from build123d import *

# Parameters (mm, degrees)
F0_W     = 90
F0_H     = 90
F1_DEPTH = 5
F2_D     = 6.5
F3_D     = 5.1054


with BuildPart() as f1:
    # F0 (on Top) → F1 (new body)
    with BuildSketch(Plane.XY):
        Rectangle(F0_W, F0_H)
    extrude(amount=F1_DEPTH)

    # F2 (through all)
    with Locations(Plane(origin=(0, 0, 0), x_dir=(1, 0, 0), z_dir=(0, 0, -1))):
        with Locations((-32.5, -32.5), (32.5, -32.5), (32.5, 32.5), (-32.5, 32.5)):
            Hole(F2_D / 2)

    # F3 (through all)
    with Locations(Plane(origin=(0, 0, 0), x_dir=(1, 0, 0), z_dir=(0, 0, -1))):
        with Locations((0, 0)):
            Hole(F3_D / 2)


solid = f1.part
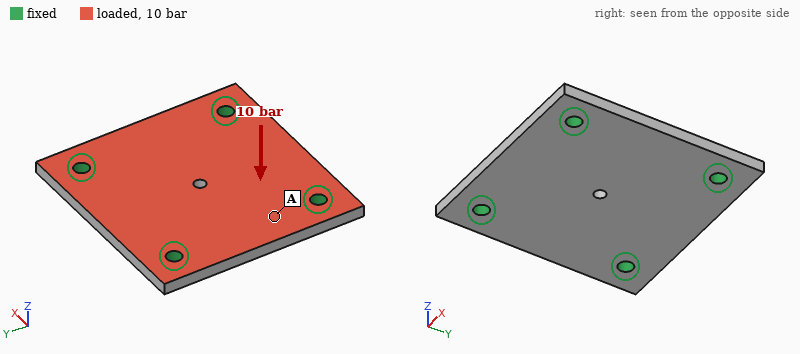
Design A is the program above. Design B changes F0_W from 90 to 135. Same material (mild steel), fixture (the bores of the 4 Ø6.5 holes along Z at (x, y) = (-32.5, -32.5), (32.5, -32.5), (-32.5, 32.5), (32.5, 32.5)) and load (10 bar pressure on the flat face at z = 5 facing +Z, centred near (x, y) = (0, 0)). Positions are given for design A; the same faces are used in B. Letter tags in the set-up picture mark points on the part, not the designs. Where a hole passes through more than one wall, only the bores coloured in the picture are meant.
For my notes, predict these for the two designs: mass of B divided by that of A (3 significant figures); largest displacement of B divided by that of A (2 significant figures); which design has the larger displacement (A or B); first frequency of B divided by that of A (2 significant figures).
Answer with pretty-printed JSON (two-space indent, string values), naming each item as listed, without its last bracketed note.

{
  "mass of B divided by that of A": "1.51",
  "largest displacement of B divided by that of A": "2.5",
  "which design has the larger displacement": "B",
  "first frequency of B divided by that of A": "0.63"
}
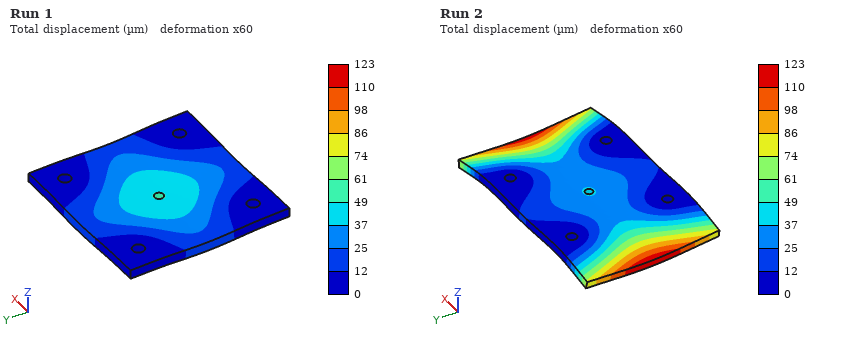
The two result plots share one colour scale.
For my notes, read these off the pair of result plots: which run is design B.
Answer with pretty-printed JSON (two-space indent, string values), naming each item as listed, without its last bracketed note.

{
  "which run is design B": "Run 2"
}
